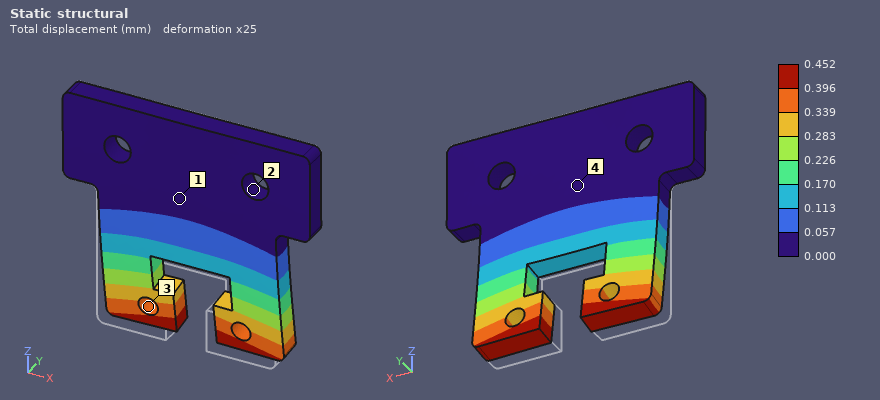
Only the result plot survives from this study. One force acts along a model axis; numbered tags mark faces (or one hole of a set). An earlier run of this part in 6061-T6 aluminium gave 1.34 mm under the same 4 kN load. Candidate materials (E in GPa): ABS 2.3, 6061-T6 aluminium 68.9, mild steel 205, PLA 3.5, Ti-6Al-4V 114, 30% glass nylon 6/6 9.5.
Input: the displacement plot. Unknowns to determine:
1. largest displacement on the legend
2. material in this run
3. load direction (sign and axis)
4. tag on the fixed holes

0.452 mm
mild steel
+Y
2
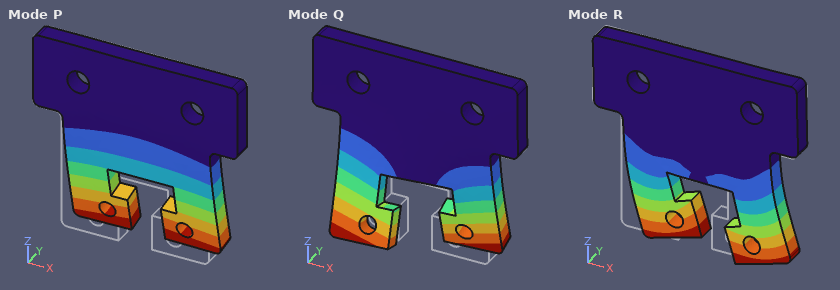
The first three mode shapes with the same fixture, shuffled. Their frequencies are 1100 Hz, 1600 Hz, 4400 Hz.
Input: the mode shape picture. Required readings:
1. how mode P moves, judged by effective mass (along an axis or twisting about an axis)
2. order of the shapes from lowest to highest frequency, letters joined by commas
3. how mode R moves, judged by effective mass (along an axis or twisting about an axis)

along Y
P, Q, R
along X
